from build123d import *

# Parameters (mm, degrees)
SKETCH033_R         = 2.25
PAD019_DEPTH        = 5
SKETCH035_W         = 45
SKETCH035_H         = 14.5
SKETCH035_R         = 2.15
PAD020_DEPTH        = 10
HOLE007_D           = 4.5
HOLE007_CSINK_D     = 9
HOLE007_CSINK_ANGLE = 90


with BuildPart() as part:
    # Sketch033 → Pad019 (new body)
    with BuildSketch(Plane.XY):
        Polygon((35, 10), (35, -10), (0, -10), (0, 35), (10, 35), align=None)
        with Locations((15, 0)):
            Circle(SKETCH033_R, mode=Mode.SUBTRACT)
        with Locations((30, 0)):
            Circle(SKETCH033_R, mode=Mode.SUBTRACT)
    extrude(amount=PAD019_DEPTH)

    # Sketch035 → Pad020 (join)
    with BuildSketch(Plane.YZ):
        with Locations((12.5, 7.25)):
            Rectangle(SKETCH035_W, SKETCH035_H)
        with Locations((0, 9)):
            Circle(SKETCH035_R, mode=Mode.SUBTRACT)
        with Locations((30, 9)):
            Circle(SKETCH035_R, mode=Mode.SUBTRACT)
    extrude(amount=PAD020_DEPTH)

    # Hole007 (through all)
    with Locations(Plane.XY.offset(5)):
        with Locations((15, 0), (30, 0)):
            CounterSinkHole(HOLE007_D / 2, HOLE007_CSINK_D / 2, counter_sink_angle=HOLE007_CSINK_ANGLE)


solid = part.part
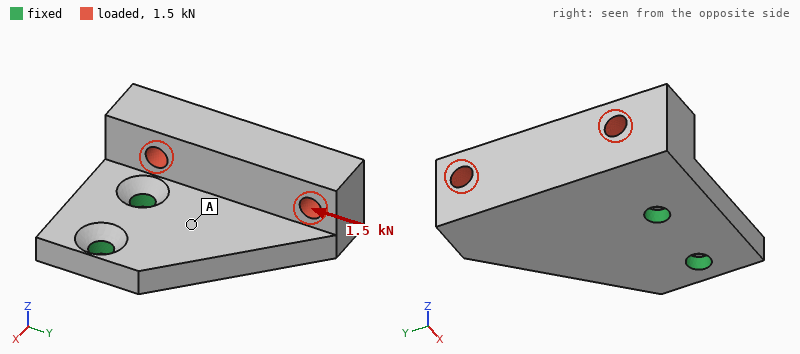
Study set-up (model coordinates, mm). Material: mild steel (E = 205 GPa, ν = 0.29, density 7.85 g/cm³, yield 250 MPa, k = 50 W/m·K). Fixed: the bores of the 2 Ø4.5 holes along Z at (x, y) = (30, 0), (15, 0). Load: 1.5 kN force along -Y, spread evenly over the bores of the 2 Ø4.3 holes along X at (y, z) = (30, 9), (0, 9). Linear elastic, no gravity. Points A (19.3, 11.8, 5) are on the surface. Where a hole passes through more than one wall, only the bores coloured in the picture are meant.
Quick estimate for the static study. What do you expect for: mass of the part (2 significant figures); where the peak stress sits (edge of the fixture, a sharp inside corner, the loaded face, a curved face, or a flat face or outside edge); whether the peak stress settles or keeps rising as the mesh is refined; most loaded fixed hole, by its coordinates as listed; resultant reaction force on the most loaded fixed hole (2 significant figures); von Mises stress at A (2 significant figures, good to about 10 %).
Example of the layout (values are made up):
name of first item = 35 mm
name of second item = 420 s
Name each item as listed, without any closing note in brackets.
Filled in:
mass of the part = 79 g
where the peak stress sits = edge of the fixture
whether the peak stress settles or keeps rising as the mesh is refined = keeps rising
most loaded fixed hole, by its coordinates as listed = (15, 0)
resultant reaction force on the most loaded fixed hole = 2.1 kN
von Mises stress at A = 26 MPa
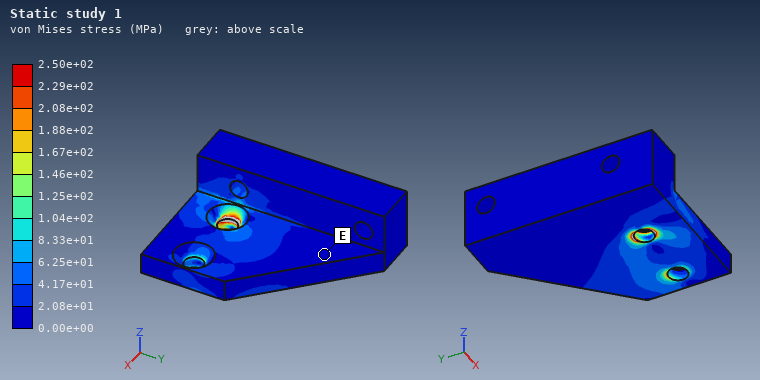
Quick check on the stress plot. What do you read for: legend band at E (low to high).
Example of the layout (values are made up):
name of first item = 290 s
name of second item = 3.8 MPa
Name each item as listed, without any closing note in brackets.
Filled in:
legend band at E = 0.00e+00 to 2.08e+01 MPa
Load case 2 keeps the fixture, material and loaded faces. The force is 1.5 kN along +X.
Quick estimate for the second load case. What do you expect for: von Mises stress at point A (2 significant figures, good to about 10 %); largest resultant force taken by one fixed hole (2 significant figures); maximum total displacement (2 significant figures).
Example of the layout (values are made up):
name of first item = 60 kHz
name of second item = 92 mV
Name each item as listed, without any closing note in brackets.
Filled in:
von Mises stress at point A = 59 MPa
largest resultant force taken by one fixed hole = 1.6 kN
maximum total displacement = 42 µm
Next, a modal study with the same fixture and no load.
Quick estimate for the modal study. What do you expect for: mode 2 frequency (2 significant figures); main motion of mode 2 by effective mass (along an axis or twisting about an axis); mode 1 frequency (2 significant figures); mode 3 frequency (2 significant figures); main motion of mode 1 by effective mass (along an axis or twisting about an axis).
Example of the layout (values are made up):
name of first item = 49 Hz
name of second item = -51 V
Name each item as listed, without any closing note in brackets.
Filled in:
mode 2 frequency = 6000 Hz
main motion of mode 2 by effective mass = along X
mode 1 frequency = 2800 Hz
mode 3 frequency = 9600 Hz
main motion of mode 1 by effective mass = along Z
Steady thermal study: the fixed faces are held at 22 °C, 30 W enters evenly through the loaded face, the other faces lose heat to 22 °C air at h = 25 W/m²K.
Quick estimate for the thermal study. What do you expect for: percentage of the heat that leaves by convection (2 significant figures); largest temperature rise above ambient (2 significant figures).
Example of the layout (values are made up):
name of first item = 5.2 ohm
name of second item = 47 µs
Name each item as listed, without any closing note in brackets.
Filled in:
percentage of the heat that leaves by convection = 13 %
largest temperature rise above ambient = 78 K
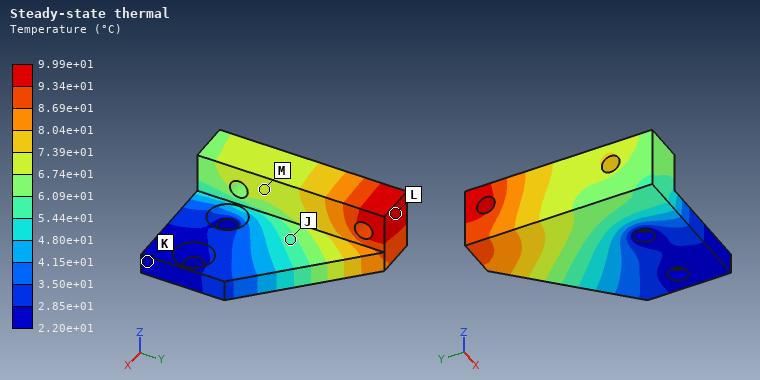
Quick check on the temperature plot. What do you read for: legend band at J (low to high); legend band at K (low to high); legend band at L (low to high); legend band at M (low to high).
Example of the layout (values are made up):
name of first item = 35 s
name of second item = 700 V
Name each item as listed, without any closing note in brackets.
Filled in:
legend band at J = 5.44e+01 to 6.09e+01 °C
legend band at K = 2.20e+01 to 2.85e+01 °C
legend band at L = 9.34e+01 to 9.99e+01 °C
legend band at M = 6.74e+01 to 7.39e+01 °C
